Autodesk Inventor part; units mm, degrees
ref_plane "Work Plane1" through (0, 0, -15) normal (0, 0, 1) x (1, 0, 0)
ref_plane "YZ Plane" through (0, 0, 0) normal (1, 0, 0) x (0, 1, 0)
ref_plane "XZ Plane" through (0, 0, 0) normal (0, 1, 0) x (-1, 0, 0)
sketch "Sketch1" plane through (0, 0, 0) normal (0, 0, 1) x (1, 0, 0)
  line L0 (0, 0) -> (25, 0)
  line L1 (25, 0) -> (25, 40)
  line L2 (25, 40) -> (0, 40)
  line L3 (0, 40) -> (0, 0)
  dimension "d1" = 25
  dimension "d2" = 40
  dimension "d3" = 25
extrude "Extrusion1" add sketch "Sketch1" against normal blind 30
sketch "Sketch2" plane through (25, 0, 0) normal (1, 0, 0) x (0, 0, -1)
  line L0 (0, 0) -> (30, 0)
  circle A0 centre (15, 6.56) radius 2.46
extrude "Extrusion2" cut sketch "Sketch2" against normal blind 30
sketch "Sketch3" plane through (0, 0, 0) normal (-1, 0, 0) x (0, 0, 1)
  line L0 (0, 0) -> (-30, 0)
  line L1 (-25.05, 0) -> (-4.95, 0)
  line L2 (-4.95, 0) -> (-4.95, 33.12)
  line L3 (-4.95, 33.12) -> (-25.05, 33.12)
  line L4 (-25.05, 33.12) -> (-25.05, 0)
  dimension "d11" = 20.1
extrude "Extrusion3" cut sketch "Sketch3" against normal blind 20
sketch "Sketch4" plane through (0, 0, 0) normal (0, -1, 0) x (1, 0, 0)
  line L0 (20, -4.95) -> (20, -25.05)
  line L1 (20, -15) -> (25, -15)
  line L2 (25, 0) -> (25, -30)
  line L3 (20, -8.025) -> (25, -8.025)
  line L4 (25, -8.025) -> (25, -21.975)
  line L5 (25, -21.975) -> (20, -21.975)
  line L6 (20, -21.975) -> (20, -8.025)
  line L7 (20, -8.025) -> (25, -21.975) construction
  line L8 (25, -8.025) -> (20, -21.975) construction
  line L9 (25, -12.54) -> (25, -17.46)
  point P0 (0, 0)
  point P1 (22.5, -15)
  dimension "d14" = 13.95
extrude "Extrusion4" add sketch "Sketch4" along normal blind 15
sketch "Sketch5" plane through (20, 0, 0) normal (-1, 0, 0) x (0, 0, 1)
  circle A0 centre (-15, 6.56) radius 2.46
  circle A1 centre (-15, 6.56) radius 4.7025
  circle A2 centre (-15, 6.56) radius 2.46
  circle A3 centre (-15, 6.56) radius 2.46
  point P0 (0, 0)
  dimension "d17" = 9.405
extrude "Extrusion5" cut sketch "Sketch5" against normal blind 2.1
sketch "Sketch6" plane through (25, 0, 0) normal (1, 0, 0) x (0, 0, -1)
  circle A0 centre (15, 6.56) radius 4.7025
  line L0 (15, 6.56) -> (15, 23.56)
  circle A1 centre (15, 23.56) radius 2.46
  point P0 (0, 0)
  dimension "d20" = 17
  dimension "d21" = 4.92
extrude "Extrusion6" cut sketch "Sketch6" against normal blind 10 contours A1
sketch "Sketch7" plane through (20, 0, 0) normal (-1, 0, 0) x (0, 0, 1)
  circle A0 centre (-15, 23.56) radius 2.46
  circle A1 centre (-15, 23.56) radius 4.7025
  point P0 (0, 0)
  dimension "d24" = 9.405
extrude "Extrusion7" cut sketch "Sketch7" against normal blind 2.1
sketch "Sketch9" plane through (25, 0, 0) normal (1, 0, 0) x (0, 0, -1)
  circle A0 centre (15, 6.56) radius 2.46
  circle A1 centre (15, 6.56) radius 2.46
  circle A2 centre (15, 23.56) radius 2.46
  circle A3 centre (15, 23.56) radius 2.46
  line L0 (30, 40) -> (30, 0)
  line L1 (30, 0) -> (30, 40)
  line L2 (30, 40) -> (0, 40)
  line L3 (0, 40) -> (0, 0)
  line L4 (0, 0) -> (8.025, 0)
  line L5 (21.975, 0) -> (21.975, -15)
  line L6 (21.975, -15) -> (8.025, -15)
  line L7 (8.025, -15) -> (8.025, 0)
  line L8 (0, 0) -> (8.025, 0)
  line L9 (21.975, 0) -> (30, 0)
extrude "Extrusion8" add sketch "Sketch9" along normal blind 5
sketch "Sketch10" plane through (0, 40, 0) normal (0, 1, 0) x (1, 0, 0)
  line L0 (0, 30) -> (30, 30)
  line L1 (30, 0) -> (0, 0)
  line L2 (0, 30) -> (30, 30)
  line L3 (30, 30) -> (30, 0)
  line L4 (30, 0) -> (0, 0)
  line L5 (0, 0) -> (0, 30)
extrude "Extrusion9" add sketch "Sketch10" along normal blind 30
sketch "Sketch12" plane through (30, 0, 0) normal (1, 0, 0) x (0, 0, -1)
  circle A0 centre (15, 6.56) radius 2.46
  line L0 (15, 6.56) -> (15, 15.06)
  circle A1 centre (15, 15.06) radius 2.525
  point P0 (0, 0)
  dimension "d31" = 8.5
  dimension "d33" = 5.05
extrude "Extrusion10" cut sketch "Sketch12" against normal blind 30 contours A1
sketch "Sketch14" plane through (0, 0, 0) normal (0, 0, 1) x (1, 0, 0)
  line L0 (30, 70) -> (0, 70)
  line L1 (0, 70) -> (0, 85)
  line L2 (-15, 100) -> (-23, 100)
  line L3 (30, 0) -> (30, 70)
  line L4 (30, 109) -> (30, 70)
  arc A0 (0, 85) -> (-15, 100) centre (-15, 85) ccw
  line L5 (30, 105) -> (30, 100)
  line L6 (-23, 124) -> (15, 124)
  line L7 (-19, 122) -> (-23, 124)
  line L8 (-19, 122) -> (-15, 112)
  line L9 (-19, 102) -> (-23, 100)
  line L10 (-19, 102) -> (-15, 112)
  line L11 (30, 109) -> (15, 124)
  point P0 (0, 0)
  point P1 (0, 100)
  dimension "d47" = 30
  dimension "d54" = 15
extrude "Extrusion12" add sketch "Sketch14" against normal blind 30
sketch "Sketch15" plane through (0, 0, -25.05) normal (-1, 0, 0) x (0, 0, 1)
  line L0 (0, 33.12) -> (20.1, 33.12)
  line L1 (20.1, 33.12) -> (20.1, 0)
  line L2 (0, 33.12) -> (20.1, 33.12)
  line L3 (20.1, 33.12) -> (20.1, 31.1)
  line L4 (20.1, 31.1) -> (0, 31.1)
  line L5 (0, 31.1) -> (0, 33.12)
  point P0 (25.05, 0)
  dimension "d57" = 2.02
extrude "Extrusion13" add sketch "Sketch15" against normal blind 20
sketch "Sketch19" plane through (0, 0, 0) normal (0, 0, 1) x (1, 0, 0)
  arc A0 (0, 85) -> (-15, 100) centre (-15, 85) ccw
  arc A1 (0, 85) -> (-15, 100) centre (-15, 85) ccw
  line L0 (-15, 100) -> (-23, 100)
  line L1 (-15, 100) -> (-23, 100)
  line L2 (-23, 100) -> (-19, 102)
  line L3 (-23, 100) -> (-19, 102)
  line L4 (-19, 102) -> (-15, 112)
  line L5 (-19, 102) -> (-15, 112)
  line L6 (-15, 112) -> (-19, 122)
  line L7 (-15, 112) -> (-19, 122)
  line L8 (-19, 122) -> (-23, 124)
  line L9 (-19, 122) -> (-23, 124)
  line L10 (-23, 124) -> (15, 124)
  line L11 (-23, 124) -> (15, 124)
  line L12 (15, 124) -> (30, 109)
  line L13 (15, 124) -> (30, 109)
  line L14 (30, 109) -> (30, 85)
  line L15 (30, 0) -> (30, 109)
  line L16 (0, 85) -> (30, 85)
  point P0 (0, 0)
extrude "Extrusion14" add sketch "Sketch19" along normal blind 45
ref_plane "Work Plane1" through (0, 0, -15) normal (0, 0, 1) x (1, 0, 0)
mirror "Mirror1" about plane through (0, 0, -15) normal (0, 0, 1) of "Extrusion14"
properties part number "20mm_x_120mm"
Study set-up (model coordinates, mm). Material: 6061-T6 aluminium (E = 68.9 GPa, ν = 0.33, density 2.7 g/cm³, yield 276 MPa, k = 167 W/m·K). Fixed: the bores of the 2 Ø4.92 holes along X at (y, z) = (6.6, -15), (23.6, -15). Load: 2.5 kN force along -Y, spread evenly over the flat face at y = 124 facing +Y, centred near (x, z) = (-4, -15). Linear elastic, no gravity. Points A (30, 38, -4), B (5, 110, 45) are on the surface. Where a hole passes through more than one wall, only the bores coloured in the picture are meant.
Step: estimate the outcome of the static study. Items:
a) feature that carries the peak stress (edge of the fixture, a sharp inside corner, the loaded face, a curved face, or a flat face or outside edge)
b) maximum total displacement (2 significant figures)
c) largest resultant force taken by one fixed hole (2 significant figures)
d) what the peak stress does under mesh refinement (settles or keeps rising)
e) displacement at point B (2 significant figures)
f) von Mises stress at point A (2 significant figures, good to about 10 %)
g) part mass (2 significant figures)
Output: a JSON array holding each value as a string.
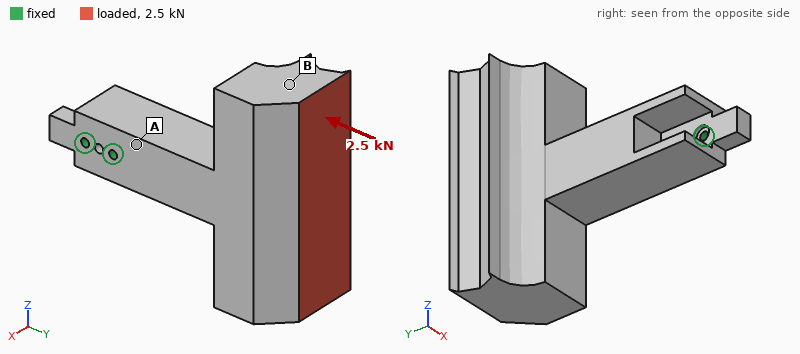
["edge of the fixture", "0.23 mm", "3.4 kN", "keeps rising", "0.18 mm", "12 MPa", "670 g"]
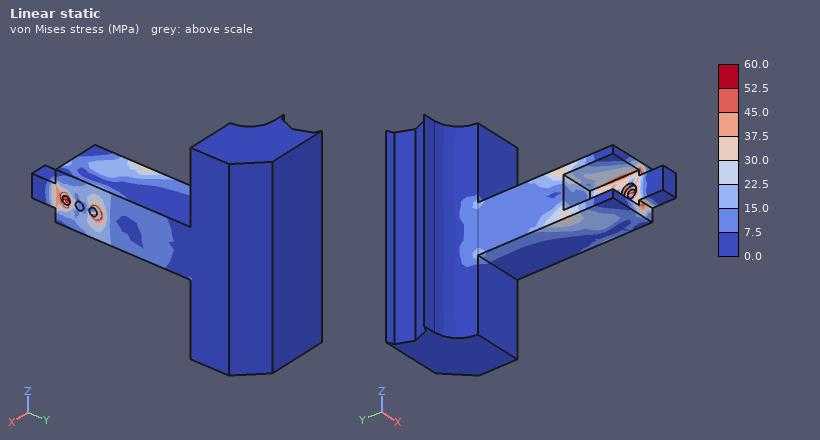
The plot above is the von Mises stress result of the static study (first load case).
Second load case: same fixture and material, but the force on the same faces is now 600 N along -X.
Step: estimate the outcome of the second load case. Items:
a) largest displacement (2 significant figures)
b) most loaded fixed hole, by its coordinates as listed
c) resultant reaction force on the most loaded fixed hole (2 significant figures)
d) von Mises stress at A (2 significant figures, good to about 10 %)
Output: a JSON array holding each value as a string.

["0.19 mm", "(23.6, -15)", "3.0 kN", "14 MPa"]
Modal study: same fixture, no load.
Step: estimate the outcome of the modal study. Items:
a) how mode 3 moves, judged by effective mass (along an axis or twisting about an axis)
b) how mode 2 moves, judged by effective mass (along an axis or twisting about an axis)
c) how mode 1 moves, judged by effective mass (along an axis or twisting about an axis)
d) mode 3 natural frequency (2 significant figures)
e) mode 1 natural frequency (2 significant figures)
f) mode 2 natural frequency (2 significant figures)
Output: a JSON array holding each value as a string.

["twisting about Y", "along Z", "along X", "750 Hz", "490 Hz", "530 Hz"]
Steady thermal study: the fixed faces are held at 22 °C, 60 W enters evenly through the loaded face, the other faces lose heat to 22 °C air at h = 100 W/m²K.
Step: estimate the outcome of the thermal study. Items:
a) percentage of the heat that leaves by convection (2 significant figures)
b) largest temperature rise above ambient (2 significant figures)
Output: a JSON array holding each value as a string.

["65 %", "20 K"]
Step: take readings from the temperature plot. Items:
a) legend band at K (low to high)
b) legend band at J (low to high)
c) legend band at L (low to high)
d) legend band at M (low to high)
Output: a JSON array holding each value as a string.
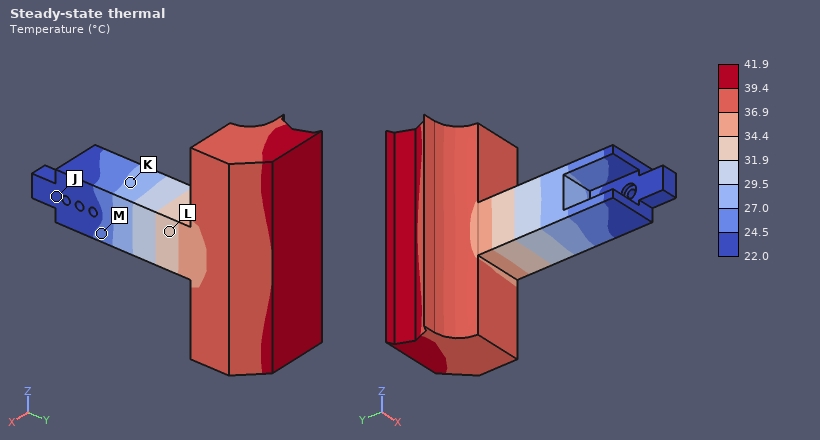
["27.0 to 29.5 °C", "22.0 to 24.5 °C", "31.9 to 34.4 °C", "24.5 to 27.0 °C"]
